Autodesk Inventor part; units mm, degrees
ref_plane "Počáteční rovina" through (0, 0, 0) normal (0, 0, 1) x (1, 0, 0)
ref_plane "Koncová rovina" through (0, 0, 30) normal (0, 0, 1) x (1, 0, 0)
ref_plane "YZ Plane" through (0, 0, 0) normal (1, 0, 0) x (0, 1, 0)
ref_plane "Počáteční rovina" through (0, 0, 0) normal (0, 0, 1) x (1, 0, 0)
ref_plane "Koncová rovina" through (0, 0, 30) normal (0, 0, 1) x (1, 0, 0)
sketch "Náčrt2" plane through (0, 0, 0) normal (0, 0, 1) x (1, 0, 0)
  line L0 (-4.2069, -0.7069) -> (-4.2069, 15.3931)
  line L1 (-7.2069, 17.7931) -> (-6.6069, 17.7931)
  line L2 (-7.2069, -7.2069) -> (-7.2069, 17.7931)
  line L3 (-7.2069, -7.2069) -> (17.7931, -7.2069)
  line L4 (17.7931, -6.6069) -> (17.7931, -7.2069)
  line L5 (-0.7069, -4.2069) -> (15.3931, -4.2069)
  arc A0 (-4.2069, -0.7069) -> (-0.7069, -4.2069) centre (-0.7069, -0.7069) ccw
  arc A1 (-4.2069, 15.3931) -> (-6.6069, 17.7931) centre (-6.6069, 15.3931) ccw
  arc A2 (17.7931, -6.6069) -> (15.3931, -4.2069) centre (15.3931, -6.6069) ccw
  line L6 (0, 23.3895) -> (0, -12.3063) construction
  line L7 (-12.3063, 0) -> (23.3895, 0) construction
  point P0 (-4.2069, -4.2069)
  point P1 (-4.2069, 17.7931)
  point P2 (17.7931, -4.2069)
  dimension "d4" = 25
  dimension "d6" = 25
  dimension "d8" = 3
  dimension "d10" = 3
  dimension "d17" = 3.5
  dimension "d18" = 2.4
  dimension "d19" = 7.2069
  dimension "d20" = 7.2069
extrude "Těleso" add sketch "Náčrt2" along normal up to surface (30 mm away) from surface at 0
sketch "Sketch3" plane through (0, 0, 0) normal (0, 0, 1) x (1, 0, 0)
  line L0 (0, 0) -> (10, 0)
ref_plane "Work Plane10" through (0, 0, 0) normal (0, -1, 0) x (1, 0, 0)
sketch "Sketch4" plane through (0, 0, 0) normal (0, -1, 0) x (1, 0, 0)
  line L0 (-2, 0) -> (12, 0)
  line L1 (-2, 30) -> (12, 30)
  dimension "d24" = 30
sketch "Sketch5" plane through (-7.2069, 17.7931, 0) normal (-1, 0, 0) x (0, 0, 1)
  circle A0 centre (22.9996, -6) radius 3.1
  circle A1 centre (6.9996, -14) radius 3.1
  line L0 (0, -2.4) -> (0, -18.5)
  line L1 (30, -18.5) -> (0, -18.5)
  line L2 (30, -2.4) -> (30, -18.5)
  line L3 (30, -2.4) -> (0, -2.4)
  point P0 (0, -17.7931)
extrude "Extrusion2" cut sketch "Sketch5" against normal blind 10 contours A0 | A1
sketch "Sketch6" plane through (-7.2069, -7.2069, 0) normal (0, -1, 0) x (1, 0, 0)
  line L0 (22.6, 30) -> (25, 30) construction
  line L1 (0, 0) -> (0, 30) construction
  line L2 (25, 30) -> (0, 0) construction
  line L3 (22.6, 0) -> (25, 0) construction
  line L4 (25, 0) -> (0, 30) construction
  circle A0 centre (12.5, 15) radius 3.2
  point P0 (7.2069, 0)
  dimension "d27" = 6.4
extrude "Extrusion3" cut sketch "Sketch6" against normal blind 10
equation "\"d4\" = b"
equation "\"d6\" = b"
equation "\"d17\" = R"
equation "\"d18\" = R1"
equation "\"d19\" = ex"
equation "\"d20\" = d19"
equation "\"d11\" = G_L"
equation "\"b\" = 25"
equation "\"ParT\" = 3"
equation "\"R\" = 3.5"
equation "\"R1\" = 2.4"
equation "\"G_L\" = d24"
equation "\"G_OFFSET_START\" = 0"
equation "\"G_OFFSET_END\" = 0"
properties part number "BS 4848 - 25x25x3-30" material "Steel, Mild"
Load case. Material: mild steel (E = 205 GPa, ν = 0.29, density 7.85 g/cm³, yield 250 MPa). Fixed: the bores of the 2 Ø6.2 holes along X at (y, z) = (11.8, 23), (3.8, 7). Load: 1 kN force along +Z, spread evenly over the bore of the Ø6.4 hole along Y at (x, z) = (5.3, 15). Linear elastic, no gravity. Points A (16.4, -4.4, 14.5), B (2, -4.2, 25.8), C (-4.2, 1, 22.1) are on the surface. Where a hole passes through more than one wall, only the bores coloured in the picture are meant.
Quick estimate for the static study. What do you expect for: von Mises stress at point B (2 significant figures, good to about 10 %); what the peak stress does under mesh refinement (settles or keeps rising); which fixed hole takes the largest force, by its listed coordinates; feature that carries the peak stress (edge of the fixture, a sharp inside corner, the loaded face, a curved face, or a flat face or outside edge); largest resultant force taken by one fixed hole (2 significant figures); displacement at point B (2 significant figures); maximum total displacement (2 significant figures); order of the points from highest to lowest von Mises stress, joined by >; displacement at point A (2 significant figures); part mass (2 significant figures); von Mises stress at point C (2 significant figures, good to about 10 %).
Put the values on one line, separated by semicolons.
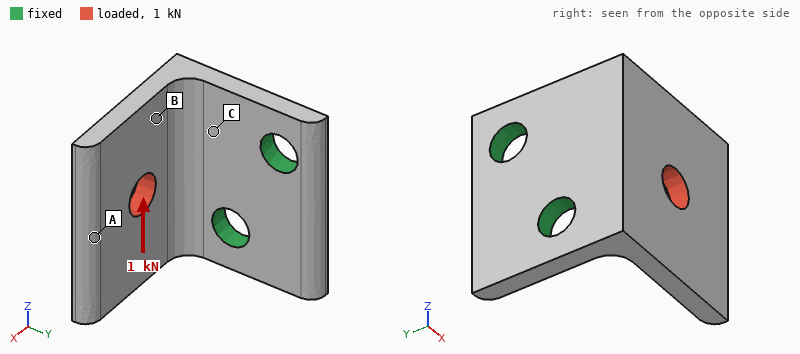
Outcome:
44 MPa; keeps rising; (3.8, 7); edge of the fixture; 1.0 kN; 38 µm; 73 µm; C > B > A; 50 µm; 31 g; 72 MPa
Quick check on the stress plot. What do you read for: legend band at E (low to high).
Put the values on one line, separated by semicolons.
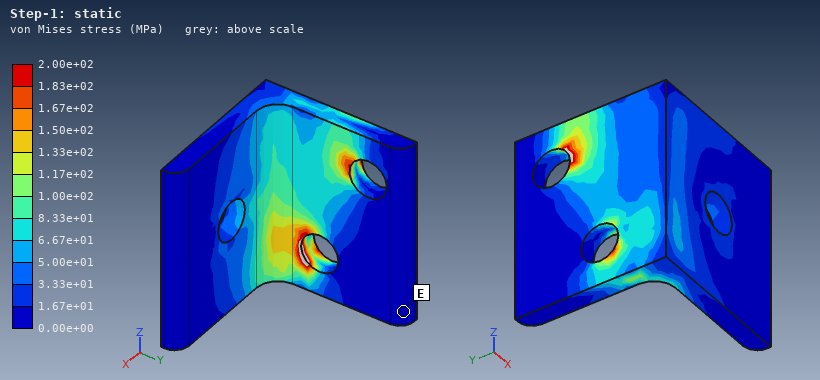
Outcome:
0.00e+00 to 1.67e+01 MPa
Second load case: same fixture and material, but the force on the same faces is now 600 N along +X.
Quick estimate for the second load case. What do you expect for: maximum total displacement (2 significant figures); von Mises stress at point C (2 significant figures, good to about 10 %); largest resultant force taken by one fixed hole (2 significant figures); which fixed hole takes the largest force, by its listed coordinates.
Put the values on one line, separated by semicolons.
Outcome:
59 µm; 43 MPa; 480 N; (3.8, 7)
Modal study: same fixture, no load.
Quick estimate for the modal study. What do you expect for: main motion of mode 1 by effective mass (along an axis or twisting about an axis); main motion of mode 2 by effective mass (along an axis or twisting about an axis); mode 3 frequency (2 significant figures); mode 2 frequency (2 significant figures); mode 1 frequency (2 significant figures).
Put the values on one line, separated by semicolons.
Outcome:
along Y; along Z; 8900 Hz; 5700 Hz; 3200 Hz
